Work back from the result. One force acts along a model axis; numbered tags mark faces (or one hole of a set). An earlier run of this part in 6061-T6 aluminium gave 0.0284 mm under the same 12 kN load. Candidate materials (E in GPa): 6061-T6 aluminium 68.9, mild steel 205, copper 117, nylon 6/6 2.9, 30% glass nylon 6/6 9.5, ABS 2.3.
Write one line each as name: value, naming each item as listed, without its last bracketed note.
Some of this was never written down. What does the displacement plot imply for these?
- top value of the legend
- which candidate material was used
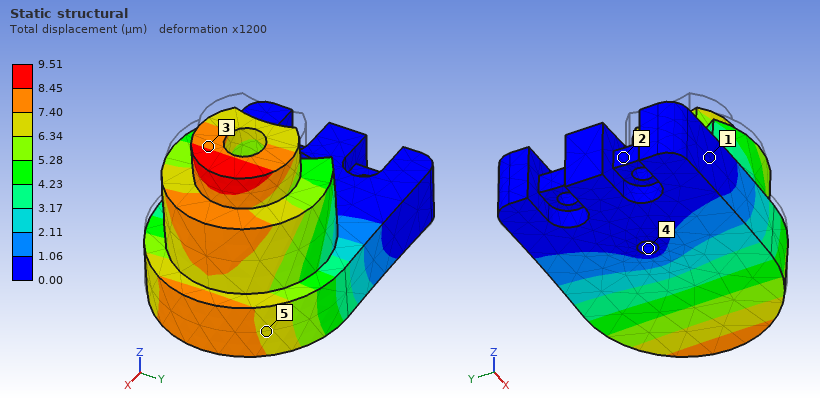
top value of the legend: 9.51 µm
which candidate material was used: mild steel
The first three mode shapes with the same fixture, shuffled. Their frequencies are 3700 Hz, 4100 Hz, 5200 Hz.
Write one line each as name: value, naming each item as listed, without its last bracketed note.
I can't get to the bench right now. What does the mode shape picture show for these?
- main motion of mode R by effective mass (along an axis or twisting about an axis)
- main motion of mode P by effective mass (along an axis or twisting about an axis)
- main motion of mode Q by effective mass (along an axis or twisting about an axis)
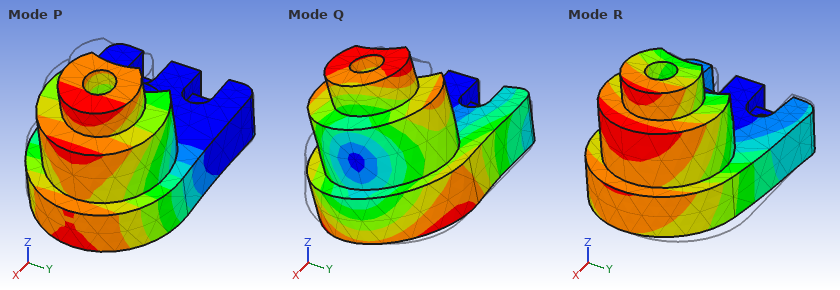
main motion of mode R by effective mass: along Y
main motion of mode P by effective mass: along Z
main motion of mode Q by effective mass: twisting about X
